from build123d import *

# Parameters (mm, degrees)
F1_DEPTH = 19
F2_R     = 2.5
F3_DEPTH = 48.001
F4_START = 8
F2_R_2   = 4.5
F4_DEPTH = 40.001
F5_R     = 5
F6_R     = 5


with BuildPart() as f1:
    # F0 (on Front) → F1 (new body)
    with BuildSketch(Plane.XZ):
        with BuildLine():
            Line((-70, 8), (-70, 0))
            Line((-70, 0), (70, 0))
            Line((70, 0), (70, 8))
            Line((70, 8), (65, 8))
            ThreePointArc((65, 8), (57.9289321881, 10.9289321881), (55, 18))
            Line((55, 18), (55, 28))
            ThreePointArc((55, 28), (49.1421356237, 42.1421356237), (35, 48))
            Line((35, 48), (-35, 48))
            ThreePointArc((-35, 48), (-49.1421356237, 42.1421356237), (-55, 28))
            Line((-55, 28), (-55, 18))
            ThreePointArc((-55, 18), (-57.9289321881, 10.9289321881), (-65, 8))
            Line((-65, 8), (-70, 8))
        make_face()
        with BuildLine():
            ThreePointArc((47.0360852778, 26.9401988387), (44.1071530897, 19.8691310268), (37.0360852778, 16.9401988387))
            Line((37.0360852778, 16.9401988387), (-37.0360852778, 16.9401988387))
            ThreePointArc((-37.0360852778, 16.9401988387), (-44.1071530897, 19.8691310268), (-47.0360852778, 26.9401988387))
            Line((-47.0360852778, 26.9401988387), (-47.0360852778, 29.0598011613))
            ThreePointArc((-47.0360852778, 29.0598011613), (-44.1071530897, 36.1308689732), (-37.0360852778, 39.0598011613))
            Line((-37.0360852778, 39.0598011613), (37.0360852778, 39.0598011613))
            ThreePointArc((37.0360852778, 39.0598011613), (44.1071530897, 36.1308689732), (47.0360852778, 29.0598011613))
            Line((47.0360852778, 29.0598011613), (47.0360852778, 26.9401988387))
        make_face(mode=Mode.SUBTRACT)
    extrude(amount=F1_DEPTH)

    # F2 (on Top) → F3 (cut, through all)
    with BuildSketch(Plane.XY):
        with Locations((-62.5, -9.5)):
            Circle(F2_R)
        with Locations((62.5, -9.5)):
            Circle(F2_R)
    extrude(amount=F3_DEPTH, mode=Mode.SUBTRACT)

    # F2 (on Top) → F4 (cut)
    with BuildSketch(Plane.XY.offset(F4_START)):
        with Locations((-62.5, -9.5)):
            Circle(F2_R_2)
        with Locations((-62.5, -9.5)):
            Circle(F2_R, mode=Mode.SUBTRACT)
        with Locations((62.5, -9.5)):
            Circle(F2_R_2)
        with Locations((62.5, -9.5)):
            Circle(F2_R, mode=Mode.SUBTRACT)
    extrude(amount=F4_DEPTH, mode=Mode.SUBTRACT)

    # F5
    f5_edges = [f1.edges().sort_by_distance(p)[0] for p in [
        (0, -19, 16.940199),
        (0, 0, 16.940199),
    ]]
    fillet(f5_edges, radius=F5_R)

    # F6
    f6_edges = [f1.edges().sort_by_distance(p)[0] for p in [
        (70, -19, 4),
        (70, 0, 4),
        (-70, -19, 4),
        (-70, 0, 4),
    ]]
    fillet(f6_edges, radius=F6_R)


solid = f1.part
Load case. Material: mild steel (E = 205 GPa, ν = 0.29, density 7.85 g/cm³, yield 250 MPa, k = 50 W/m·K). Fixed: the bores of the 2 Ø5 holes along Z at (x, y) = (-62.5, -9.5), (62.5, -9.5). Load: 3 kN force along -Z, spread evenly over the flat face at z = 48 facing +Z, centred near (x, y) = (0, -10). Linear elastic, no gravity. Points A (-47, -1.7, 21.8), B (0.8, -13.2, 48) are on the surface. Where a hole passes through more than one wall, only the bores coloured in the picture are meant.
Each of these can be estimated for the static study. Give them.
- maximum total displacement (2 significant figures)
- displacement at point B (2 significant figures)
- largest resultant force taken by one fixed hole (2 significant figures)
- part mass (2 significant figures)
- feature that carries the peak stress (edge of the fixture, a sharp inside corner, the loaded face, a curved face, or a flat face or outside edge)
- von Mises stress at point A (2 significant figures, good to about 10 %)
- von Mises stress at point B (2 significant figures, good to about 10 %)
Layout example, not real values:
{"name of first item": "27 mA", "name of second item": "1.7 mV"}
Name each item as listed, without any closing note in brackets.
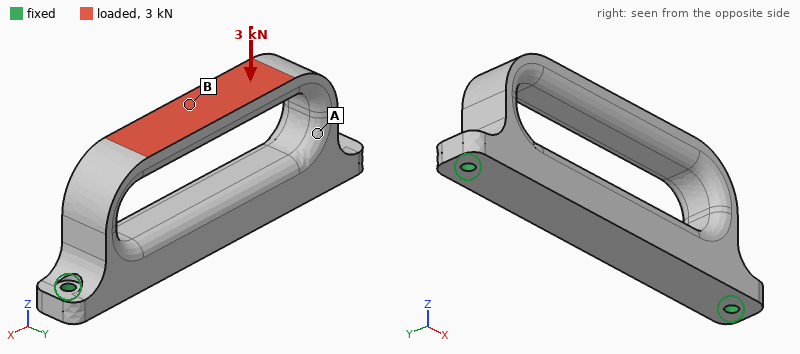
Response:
{"maximum total displacement": "75 µm", "displacement at point B": "74 µm", "largest resultant force taken by one fixed hole": "1.6 kN", "part mass": "480 g", "feature that carries the peak stress": "a curved face", "von Mises stress at point A": "21 MPa", "von Mises stress at point B": "95 MPa"}
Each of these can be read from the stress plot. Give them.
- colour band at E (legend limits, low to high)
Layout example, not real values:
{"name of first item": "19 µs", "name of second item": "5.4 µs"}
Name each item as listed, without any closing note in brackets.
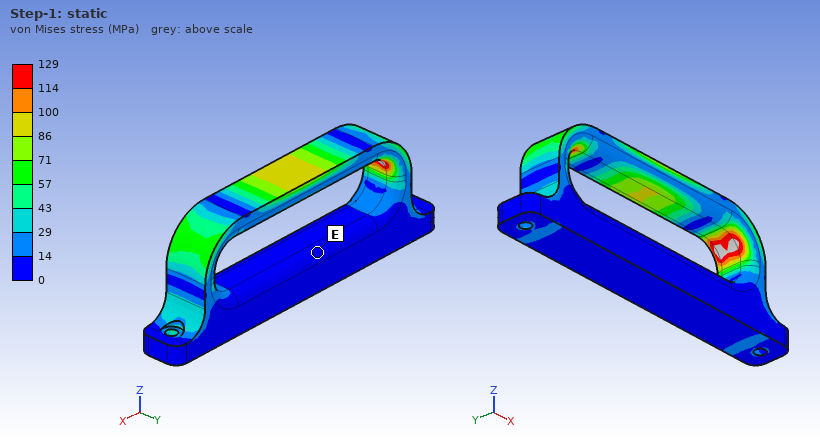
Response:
{"colour band at E": "0 to 14 MPa"}
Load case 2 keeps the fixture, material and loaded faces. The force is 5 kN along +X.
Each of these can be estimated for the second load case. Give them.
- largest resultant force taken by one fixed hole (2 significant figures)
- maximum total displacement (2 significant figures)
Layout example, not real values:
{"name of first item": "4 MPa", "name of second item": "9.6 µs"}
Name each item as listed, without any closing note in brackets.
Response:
{"largest resultant force taken by one fixed hole": "3.0 kN", "maximum total displacement": "58 µm"}
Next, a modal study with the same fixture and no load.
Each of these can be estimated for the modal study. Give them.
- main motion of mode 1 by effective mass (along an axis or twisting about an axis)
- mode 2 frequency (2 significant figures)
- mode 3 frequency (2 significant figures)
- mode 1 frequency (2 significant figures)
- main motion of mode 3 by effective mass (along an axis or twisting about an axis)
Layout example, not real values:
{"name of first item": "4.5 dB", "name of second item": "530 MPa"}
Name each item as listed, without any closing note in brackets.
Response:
{"main motion of mode 1 by effective mass": "along Y", "mode 2 frequency": "3600 Hz", "mode 3 frequency": "3900 Hz", "mode 1 frequency": "2100 Hz", "main motion of mode 3 by effective mass": "along X"}
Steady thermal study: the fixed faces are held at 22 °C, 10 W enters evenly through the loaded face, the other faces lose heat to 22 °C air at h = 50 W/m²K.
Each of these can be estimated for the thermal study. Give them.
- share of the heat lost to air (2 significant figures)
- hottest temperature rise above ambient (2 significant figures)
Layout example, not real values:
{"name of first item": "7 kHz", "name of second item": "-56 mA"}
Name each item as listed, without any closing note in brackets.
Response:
{"share of the heat lost to air": "58 %", "hottest temperature rise above ambient": "27 K"}
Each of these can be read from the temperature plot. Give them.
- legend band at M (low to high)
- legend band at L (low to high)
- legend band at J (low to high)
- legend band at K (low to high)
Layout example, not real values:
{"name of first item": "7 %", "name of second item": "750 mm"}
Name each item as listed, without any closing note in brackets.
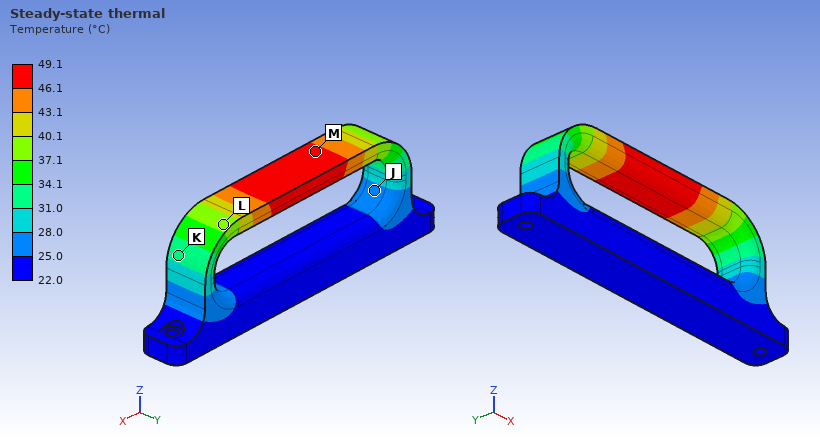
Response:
{"legend band at M": "46.1 to 49.1 °C", "legend band at L": "37.1 to 40.1 °C", "legend band at J": "25.0 to 28.0 °C", "legend band at K": "31.0 to 34.1 °C"}
